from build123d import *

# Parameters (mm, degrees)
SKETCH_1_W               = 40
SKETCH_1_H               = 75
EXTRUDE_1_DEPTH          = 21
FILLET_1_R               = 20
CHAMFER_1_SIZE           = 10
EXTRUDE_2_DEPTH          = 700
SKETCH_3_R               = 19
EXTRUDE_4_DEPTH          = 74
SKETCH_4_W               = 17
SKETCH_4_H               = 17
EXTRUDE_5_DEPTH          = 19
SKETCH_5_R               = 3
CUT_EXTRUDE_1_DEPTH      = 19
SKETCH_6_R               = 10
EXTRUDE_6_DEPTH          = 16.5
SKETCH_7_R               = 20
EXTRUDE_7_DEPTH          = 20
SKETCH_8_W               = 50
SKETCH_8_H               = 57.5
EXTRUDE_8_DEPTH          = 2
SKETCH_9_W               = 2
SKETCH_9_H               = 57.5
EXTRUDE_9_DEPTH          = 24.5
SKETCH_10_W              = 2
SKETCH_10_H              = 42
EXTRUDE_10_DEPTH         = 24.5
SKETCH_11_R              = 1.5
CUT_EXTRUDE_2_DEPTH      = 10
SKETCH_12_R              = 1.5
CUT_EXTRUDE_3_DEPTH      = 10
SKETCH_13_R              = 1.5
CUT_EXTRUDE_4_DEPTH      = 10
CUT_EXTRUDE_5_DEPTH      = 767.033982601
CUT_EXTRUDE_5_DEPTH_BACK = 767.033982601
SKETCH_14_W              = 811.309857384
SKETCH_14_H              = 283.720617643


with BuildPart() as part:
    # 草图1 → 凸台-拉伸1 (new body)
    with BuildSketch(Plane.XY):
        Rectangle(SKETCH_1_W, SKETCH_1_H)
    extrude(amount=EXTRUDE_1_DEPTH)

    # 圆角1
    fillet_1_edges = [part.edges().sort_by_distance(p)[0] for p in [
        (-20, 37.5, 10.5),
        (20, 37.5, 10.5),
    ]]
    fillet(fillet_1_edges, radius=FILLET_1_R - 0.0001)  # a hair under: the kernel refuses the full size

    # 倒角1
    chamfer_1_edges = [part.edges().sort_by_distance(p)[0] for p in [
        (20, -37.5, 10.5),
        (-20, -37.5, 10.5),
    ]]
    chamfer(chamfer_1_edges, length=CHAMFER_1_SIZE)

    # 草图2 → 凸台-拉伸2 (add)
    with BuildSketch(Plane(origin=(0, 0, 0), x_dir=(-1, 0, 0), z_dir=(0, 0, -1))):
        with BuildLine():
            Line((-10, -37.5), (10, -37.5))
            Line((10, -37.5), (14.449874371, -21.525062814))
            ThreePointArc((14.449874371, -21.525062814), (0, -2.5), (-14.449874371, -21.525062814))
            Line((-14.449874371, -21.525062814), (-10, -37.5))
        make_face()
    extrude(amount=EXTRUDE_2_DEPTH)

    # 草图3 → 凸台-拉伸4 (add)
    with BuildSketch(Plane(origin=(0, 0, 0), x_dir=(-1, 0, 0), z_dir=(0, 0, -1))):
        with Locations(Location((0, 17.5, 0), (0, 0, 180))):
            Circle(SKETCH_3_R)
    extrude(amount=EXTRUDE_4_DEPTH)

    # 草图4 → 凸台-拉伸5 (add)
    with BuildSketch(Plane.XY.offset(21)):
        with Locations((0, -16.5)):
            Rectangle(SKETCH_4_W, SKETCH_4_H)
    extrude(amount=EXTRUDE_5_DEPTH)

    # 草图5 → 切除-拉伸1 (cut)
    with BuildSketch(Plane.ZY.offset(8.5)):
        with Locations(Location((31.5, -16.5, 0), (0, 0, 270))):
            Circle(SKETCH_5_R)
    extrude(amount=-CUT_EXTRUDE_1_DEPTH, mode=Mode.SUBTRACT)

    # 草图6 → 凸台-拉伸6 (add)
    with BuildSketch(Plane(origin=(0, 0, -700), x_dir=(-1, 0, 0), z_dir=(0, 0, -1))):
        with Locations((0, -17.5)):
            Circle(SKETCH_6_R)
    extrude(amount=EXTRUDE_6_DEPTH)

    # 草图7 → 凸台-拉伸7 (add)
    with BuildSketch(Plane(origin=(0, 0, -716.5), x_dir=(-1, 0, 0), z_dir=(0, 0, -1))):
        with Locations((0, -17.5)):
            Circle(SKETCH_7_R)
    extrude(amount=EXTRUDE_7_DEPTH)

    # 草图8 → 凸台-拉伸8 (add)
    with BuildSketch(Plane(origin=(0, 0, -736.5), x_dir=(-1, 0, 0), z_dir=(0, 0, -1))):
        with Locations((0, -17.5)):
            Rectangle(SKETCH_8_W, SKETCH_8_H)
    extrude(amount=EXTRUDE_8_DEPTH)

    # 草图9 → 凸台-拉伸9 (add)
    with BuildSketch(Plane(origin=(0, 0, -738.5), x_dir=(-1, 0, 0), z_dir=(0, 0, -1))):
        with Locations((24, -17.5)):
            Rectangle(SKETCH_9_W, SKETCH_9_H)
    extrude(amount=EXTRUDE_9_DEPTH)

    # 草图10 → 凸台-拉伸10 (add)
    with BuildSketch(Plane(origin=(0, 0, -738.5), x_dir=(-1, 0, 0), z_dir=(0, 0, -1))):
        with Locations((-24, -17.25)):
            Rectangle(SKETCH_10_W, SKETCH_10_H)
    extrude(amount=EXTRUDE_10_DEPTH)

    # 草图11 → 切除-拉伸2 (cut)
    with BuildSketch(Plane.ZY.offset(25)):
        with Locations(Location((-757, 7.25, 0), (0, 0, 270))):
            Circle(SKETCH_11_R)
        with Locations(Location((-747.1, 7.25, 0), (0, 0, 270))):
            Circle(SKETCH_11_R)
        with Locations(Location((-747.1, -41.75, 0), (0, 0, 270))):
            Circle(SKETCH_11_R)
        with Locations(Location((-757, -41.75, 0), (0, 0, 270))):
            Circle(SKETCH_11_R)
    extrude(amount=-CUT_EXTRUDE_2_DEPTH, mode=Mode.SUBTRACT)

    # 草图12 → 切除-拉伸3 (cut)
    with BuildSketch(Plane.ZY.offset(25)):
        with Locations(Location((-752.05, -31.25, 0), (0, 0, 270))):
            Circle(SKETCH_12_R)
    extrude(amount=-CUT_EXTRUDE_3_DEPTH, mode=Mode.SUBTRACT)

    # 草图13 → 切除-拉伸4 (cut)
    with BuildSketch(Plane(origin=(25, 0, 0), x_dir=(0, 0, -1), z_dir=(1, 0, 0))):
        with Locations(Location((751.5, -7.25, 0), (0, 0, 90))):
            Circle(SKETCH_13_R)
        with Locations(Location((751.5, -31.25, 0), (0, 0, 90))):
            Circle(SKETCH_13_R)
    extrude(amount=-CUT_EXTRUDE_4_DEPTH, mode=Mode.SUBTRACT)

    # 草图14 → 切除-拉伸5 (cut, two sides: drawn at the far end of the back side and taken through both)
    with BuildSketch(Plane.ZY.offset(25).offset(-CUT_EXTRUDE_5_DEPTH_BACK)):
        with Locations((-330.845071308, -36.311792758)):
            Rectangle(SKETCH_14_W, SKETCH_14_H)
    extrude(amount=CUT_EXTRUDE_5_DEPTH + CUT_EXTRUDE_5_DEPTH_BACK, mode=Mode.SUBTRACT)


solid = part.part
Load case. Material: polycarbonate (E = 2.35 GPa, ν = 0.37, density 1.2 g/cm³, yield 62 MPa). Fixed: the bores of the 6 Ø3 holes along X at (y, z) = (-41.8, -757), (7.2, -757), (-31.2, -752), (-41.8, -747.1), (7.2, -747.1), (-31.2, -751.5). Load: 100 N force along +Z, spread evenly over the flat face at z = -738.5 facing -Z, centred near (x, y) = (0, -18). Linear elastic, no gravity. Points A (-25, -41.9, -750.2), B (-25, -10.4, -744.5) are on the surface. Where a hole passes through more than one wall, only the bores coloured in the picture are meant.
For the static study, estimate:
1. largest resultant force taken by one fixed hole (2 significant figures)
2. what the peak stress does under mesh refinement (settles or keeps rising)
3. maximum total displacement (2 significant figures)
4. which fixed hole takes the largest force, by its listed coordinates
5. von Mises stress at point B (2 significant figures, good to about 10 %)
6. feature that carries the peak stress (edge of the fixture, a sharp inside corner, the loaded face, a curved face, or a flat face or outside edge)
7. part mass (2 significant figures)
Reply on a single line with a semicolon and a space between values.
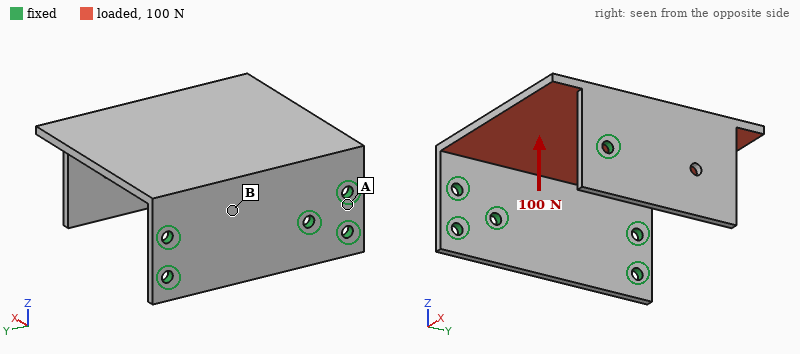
60 N; keeps rising; 0.91 mm; (-31.2, -751.5); 3.7 MPa; edge of the fixture; 13 g
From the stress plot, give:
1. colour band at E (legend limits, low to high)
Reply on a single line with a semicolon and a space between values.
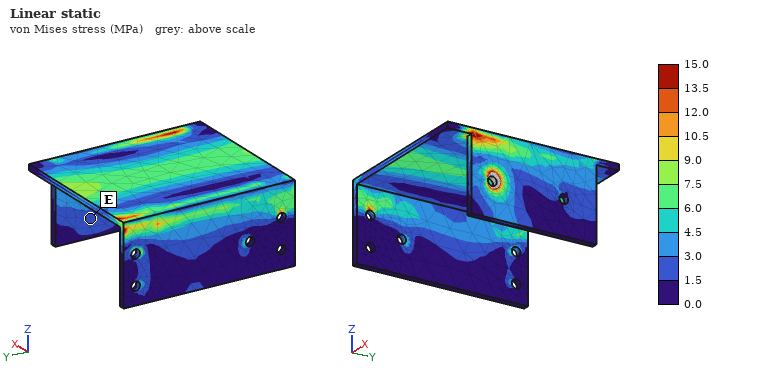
1.5 to 3.0 MPa
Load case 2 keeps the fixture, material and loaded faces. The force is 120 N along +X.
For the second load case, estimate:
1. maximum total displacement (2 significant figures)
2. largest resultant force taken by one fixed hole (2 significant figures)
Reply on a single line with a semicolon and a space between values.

0.44 mm; 49 N
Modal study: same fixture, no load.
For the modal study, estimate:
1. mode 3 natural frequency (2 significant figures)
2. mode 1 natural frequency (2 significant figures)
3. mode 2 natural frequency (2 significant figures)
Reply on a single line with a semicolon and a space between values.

1000 Hz; 730 Hz; 800 Hz
